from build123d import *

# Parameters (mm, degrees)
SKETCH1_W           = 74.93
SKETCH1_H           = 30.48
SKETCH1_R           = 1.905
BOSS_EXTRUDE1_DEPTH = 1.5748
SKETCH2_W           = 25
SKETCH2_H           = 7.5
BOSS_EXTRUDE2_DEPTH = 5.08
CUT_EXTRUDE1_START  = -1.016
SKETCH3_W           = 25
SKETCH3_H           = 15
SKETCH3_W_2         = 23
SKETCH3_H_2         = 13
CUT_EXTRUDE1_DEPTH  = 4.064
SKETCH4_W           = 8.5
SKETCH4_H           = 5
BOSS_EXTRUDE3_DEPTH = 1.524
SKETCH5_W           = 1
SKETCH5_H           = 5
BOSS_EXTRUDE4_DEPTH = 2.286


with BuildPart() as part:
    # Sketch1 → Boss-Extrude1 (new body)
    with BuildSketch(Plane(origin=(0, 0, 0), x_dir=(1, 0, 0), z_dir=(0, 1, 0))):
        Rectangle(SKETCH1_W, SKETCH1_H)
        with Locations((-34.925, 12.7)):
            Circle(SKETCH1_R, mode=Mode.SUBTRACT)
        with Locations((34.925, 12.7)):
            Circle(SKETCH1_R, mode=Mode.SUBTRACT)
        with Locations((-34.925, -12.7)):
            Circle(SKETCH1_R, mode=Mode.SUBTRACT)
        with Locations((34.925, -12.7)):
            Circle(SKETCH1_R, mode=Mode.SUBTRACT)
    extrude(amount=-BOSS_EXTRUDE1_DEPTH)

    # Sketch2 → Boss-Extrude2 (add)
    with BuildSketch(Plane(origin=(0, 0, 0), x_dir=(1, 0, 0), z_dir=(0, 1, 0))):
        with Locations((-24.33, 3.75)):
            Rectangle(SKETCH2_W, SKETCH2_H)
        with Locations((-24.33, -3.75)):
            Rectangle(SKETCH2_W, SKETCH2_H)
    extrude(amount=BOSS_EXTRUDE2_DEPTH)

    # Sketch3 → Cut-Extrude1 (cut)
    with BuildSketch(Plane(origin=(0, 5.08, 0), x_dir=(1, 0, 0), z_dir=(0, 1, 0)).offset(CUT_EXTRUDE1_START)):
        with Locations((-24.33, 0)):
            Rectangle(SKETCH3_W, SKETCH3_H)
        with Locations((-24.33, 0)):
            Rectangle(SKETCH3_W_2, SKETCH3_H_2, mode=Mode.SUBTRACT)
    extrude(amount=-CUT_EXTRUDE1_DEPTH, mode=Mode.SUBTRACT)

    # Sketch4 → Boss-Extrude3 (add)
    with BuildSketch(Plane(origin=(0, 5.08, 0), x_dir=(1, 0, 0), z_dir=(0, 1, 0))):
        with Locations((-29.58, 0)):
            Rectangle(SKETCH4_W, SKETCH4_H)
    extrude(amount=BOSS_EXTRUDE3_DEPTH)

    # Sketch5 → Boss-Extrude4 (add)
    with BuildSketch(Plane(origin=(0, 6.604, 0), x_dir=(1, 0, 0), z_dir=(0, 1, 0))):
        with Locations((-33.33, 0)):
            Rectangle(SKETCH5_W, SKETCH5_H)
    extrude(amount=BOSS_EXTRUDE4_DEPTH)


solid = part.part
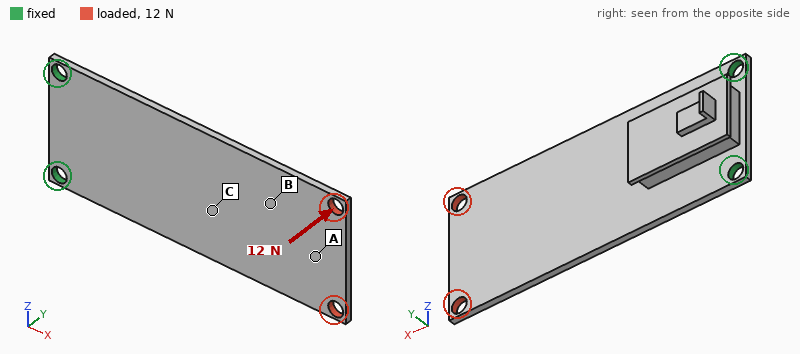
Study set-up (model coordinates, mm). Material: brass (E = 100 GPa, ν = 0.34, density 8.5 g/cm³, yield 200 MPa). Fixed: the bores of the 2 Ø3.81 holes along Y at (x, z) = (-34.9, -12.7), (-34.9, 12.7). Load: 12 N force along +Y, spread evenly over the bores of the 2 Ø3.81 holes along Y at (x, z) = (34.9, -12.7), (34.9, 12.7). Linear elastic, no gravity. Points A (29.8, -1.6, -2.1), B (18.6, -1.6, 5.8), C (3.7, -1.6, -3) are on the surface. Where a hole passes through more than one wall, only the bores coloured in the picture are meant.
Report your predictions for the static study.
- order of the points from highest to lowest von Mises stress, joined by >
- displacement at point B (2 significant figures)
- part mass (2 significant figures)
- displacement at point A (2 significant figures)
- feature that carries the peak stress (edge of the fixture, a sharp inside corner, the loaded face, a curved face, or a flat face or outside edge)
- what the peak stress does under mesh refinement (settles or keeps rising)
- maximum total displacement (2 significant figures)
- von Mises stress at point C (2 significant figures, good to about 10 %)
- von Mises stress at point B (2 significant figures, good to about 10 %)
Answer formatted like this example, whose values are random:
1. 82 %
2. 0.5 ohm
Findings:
1. C > B > A
2. 0.42 mm
3. 44 g
4. 0.61 mm
5. edge of the fixture
6. keeps rising
7. 0.74 mm
8. 27 MPa
9. 15 MPa
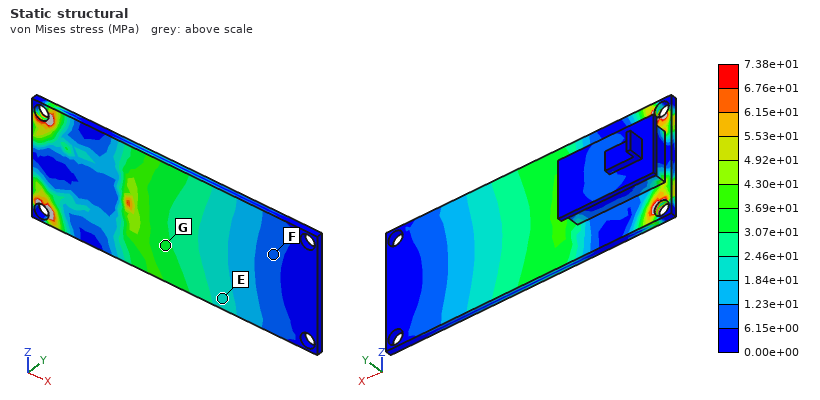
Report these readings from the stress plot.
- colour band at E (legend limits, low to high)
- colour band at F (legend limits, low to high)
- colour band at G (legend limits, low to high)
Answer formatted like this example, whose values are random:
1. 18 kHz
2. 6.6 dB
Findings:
1. 1.84e+01 to 2.46e+01 MPa
2. 6.15e+00 to 1.23e+01 MPa
3. 3.07e+01 to 3.69e+01 MPa
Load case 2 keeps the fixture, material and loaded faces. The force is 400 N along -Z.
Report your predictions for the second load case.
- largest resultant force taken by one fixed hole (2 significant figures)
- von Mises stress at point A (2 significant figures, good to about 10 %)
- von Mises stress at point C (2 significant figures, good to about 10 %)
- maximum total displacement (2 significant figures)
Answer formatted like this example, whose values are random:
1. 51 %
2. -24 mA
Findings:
1. 1.1 kN
2. 20 MPa
3. 23 MPa
4. 0.14 mm
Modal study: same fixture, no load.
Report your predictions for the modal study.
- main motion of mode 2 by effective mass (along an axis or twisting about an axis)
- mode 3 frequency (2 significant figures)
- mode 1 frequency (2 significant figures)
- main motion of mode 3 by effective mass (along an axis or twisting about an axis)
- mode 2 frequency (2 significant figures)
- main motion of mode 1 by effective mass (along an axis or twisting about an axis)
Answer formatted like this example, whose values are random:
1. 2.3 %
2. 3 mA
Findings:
1. along Y
2. 1200 Hz
3. 250 Hz
4. twisting about X
5. 1100 Hz
6. along Y
